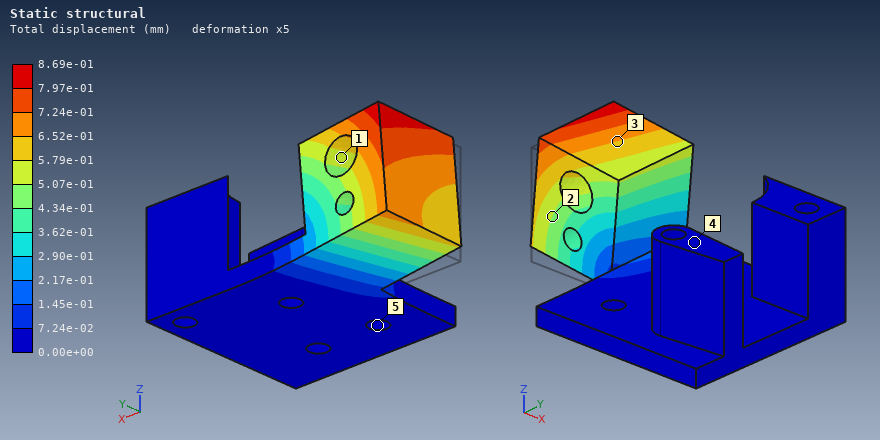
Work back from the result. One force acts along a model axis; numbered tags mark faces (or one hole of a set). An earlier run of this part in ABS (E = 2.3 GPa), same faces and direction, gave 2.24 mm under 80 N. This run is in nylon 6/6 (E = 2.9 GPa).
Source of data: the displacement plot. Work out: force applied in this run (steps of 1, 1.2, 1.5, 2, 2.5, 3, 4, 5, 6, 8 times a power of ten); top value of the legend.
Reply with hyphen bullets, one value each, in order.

- 40 N
- 8.69e-01 mm
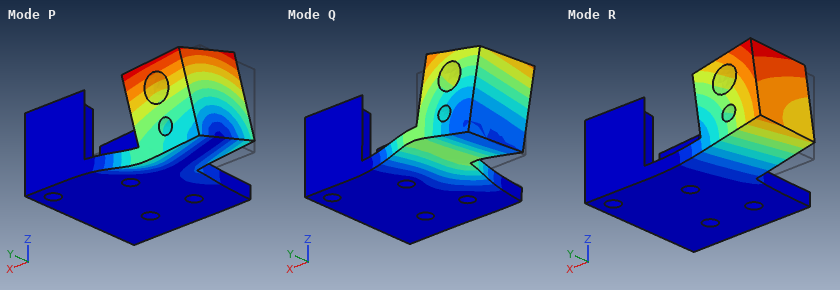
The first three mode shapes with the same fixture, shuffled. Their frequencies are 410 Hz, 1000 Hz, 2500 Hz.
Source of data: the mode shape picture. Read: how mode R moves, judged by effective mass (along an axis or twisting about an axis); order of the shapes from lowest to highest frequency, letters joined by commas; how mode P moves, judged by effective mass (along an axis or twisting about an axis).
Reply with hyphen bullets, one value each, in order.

- along Z
- R, P, Q
- along Y
